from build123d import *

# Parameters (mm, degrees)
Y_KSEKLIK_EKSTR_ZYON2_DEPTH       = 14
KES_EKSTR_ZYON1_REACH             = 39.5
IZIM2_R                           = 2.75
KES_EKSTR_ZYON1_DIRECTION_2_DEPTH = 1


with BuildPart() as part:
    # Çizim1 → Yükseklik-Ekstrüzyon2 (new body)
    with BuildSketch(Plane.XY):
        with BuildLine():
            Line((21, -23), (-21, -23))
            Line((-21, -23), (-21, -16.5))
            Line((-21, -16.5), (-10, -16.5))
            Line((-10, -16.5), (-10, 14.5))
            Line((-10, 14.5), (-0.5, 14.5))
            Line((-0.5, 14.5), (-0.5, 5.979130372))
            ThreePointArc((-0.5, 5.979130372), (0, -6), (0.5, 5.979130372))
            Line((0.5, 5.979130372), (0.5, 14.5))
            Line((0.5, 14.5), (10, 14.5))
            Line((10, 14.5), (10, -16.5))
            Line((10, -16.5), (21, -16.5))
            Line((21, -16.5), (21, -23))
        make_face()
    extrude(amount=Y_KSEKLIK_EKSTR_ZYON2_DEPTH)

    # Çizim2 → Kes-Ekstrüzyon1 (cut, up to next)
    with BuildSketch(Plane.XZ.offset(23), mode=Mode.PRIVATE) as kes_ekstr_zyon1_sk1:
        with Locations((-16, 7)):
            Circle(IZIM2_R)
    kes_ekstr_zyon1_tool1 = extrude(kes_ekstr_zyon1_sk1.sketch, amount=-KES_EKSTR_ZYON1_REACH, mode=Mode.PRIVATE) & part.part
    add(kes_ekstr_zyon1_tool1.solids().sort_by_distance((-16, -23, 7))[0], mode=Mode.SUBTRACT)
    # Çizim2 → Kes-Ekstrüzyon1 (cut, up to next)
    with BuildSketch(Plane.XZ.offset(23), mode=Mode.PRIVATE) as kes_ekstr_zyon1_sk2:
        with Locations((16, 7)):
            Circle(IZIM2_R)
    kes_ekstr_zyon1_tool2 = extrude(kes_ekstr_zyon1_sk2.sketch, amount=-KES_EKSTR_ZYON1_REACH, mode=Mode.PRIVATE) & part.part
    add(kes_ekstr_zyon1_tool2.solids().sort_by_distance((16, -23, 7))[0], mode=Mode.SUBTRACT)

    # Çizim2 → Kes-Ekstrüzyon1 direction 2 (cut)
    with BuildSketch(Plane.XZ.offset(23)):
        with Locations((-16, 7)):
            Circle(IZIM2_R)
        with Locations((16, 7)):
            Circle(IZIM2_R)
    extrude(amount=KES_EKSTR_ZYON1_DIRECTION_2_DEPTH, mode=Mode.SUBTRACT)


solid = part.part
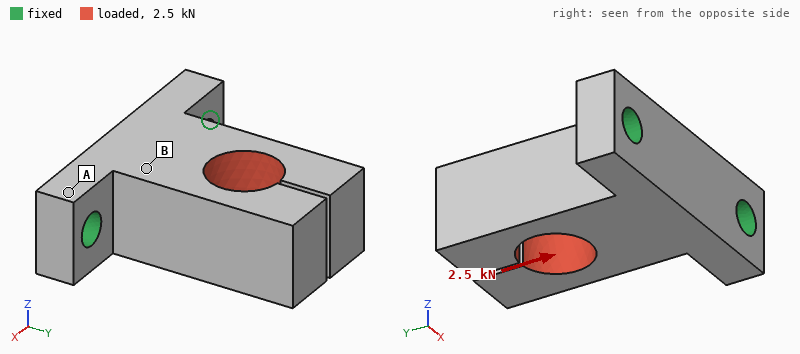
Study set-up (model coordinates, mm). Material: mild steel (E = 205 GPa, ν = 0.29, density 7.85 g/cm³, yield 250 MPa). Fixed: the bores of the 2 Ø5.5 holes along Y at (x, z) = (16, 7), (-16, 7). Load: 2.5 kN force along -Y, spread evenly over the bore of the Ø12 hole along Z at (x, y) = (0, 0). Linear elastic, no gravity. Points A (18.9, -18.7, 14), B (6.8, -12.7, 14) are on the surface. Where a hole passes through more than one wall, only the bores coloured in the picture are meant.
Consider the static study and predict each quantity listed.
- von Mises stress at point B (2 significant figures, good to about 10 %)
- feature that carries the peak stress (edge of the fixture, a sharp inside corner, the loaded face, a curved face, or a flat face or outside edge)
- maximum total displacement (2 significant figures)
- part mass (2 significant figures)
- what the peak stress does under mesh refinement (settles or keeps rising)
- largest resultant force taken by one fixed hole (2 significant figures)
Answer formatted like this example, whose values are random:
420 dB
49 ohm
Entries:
17 MPa
edge of the fixture
23 µm
82 g
keeps rising
1.3 kN
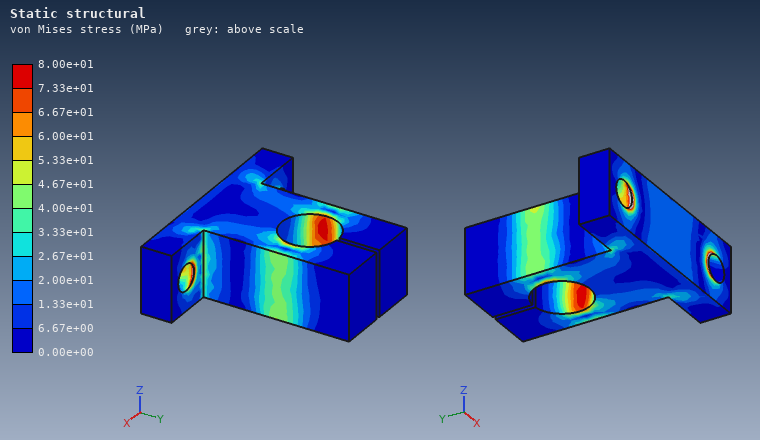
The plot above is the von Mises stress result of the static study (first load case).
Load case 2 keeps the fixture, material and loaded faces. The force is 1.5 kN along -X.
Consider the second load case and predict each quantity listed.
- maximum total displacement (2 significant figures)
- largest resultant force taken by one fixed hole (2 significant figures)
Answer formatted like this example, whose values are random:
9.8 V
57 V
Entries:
27 µm
1.4 kN
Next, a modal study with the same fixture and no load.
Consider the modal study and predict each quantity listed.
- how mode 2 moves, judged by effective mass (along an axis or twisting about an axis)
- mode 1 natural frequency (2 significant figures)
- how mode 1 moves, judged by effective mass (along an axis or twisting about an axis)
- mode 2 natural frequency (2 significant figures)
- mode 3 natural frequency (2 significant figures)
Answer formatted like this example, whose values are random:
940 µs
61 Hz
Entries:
along X
4500 Hz
along Z
5200 Hz
5600 Hz
